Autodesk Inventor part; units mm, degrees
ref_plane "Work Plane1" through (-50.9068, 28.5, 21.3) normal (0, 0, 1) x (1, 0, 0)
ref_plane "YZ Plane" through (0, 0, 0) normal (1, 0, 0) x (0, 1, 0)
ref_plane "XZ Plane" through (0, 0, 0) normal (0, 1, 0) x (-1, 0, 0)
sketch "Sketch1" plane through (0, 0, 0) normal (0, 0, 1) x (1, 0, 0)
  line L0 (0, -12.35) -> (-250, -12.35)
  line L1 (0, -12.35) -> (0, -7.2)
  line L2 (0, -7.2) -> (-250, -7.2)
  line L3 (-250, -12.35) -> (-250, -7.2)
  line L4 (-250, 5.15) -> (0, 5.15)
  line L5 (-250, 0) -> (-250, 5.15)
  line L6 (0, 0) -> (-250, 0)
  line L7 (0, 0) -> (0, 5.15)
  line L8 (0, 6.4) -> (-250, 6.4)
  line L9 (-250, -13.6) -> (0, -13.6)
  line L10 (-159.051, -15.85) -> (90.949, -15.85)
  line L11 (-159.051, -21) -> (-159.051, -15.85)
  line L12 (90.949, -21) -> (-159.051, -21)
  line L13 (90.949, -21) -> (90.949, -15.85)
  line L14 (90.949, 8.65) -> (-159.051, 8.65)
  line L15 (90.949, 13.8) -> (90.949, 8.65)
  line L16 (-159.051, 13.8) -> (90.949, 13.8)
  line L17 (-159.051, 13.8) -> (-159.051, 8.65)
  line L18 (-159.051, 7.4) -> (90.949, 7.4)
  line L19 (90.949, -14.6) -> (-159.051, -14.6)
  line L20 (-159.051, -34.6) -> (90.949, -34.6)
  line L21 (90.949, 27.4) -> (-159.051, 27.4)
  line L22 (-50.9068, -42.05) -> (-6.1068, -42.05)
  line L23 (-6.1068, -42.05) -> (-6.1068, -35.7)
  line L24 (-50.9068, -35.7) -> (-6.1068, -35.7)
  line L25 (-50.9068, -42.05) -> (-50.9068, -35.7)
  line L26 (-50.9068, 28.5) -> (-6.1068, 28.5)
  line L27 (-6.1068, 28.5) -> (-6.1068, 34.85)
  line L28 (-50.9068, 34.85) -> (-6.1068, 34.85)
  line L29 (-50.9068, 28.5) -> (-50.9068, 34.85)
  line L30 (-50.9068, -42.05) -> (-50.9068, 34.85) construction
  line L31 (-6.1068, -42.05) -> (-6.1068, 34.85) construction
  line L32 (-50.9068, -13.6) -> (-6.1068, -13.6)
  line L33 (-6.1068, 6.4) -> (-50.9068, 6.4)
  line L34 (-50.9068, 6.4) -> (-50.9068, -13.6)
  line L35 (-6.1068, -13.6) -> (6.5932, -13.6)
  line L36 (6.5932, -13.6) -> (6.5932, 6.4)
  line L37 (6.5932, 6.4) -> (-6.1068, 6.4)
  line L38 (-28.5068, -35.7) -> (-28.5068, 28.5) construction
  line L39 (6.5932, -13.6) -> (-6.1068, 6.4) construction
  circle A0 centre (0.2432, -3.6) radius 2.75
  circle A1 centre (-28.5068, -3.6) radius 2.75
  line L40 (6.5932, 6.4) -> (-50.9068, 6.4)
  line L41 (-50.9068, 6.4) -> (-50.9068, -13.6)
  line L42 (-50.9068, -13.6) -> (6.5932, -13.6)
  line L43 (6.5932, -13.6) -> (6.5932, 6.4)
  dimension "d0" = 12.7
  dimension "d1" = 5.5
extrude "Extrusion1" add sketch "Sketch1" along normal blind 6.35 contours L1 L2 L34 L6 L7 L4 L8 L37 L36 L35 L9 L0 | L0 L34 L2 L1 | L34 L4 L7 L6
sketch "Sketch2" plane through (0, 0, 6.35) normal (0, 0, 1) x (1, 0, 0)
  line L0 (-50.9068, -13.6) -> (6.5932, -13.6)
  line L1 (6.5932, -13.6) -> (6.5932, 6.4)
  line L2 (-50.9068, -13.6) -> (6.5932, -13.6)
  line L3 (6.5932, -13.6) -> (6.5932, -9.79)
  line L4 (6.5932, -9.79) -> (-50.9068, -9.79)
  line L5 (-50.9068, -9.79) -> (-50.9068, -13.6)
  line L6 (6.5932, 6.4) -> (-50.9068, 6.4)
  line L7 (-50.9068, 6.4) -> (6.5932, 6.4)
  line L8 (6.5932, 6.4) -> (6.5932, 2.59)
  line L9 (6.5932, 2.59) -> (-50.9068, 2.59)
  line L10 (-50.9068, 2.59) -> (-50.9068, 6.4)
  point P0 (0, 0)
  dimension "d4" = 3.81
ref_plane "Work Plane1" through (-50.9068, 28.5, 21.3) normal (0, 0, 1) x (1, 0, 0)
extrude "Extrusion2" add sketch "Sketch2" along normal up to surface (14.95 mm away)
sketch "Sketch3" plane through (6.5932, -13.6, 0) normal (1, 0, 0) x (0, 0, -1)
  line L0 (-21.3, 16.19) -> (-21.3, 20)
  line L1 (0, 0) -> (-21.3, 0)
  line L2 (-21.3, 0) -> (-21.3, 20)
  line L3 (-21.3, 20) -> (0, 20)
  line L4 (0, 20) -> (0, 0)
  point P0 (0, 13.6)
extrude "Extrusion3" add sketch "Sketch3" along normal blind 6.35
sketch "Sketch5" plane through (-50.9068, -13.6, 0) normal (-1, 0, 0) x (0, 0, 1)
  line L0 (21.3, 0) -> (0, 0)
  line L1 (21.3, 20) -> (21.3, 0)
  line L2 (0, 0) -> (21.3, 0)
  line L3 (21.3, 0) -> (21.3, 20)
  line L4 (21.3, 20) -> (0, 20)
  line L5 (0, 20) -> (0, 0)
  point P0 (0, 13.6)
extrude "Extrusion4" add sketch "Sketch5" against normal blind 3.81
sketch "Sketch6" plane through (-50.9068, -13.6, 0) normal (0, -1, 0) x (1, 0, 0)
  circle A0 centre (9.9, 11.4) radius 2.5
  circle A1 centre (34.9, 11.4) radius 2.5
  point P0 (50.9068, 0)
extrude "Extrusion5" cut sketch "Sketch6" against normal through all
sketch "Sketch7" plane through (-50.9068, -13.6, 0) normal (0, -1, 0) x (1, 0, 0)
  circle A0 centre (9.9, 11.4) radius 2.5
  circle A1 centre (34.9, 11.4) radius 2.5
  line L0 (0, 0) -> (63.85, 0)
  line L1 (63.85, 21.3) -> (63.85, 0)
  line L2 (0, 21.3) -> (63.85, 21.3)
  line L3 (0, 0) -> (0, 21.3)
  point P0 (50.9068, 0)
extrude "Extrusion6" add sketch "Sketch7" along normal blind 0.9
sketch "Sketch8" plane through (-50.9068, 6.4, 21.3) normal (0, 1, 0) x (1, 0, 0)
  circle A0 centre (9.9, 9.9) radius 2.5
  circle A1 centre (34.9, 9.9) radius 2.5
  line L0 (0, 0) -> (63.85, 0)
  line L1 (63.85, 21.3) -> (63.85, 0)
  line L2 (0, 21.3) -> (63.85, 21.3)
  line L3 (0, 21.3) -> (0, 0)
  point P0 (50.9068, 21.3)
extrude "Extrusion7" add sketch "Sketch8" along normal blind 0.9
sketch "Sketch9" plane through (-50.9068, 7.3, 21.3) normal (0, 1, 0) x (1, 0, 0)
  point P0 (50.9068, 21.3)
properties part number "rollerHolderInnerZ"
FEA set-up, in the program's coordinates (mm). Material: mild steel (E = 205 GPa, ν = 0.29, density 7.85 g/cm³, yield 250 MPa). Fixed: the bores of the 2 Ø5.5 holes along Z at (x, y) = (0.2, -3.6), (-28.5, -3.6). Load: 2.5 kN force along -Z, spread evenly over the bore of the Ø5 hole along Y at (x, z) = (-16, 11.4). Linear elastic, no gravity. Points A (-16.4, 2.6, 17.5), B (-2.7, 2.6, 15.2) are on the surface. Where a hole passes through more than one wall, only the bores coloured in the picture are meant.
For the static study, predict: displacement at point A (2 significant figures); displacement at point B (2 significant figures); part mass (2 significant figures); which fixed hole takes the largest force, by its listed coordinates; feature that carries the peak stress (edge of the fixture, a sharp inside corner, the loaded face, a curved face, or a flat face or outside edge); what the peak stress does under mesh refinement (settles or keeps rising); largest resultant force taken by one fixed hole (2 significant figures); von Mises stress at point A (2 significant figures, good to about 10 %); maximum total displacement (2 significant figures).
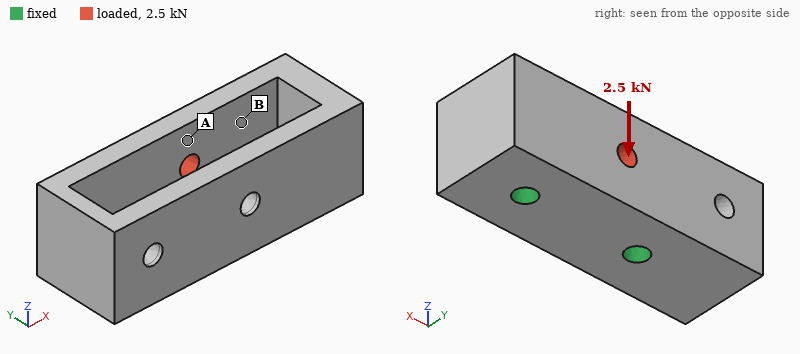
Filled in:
7.9 µm
4.9 µm
150 g
(-28.5, -3.6)
edge of the fixture
keeps rising
1.5 kN
33 MPa
10.0 µm
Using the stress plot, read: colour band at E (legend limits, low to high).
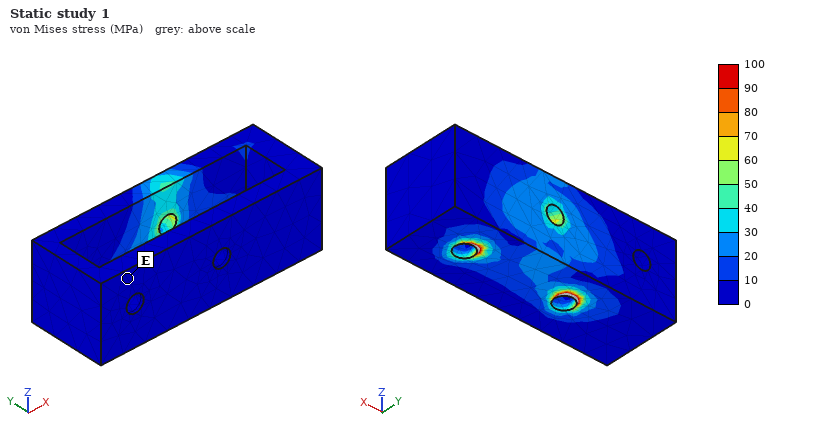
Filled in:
0 to 10 MPa
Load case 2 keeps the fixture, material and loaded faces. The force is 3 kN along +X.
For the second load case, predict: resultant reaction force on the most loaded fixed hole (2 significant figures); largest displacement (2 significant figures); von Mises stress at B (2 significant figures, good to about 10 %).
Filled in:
1.8 kN
6.1 µm
16 MPa
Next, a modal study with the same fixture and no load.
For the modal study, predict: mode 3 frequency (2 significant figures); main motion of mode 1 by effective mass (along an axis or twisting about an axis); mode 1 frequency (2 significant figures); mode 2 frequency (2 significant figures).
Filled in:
11 kHz
along Y
7700 Hz
10 kHz
